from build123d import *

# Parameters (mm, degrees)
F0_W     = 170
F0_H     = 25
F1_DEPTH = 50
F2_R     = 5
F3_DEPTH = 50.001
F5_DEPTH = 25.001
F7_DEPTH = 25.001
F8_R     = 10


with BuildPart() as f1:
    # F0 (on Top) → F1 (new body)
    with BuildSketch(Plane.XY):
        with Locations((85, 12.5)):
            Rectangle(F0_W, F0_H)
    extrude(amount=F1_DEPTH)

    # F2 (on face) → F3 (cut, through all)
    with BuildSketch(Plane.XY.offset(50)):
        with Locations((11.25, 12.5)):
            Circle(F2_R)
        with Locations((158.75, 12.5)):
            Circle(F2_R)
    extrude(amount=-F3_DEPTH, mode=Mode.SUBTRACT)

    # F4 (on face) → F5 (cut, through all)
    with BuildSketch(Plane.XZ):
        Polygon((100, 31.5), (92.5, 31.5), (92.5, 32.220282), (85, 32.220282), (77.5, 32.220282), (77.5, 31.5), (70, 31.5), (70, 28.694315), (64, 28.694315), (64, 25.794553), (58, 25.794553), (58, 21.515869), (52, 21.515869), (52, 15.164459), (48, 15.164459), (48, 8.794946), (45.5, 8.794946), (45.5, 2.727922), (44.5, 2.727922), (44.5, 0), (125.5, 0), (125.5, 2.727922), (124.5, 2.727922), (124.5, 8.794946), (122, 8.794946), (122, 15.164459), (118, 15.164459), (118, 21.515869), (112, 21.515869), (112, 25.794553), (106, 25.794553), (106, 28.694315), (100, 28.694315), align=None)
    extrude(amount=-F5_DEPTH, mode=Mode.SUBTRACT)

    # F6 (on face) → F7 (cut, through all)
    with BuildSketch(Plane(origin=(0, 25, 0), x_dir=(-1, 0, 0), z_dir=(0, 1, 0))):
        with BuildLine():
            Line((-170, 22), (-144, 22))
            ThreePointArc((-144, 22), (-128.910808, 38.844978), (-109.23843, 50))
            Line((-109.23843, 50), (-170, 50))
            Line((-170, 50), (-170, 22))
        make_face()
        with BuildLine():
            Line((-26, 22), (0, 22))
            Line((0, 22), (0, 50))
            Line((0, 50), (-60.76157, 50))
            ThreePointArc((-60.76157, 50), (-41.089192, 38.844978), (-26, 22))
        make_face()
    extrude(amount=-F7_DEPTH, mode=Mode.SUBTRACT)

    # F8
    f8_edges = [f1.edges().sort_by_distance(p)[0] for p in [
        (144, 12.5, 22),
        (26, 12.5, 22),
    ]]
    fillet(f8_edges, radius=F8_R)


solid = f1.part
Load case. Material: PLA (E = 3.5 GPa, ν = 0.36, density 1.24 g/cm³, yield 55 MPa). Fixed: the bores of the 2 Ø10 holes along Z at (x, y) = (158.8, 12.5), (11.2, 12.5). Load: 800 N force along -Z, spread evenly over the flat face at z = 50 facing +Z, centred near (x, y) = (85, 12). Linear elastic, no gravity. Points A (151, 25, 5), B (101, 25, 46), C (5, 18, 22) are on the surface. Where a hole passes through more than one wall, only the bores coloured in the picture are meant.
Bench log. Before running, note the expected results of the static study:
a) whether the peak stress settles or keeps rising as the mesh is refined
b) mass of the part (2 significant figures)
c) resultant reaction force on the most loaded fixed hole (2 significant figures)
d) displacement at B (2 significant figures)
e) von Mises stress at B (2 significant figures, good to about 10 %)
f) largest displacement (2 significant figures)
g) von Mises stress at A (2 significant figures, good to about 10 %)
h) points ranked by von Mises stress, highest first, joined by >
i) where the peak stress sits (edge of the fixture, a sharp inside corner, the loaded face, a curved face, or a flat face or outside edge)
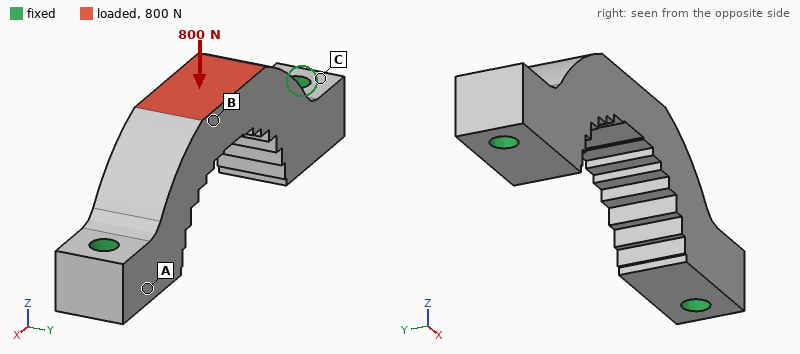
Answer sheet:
keeps rising
130 g
660 N
61 µm
1.6 MPa
72 µm
0.98 MPa
B > A > C
edge of the fixture
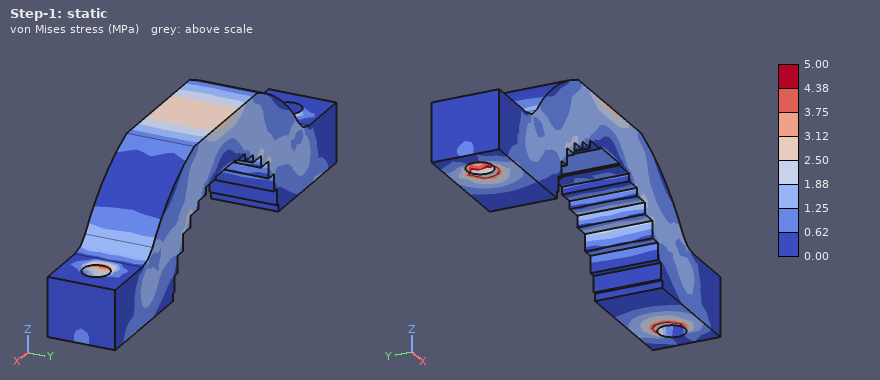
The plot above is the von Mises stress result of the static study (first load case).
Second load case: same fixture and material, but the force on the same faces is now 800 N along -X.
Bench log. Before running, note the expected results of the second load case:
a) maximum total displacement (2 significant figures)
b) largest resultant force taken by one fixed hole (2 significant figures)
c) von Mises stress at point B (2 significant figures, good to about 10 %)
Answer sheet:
27 µm
460 N
0.95 MPa
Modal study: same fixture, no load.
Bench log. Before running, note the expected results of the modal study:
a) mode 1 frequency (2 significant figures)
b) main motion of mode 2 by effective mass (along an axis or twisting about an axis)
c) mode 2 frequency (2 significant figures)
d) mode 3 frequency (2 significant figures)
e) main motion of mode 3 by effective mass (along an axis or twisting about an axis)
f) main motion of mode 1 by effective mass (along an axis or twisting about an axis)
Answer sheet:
1100 Hz
along Z
2500 Hz
2800 Hz
along X
along Y
